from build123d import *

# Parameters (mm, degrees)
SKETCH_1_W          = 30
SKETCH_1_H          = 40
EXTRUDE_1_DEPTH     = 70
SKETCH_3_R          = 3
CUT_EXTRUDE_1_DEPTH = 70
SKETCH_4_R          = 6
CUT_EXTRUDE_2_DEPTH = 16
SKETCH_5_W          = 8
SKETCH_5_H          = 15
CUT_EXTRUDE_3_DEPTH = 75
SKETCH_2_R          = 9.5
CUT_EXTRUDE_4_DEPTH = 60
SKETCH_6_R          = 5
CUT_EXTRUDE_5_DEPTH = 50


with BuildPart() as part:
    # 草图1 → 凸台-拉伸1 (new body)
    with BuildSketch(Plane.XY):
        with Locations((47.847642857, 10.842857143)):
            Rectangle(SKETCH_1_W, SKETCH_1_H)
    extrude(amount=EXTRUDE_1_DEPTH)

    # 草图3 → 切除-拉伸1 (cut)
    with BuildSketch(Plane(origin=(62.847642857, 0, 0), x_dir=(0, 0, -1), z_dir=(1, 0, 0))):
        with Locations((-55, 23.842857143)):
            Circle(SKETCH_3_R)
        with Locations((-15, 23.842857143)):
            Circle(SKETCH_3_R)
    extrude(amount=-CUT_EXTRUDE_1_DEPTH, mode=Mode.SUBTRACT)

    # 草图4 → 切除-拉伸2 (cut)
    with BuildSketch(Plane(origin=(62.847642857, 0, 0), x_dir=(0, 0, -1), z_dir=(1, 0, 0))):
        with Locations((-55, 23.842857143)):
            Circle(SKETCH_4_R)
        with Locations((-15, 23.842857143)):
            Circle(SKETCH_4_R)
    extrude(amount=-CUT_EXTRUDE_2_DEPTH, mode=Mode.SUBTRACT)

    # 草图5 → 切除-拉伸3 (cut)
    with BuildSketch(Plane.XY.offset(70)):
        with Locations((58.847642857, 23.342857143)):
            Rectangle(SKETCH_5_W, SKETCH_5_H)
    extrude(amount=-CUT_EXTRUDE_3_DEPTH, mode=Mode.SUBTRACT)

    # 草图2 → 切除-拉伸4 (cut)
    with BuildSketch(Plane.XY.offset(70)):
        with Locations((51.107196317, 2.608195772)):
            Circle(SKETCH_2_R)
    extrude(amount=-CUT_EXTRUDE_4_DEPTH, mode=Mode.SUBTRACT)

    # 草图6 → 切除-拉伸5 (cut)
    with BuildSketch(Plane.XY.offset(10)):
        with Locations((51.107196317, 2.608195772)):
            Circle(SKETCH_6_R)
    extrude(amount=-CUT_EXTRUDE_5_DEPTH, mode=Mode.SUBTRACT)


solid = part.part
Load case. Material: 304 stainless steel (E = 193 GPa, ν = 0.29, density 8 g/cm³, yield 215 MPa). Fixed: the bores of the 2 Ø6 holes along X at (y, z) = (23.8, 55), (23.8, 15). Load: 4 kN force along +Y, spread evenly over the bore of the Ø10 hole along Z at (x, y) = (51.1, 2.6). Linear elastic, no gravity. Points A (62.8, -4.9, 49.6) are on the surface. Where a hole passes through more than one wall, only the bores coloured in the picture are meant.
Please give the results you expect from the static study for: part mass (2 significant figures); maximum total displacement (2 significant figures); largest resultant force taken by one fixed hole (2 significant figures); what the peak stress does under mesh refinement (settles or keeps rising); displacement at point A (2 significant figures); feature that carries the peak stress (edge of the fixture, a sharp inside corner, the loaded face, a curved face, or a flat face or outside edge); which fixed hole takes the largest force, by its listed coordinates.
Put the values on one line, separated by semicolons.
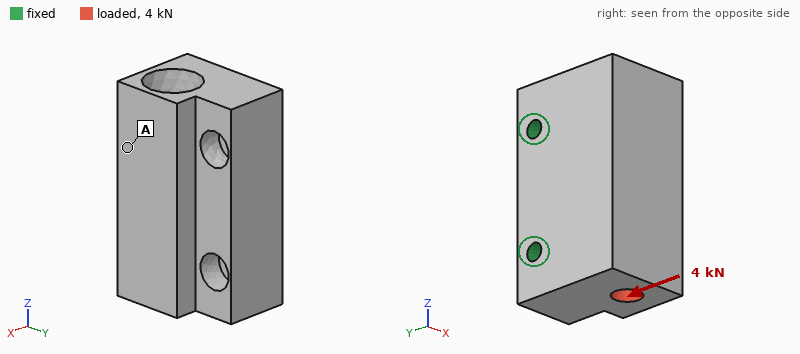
440 g; 12 µm; 4.7 kN; keeps rising; 6.0 µm; edge of the fixture; (23.8, 15)
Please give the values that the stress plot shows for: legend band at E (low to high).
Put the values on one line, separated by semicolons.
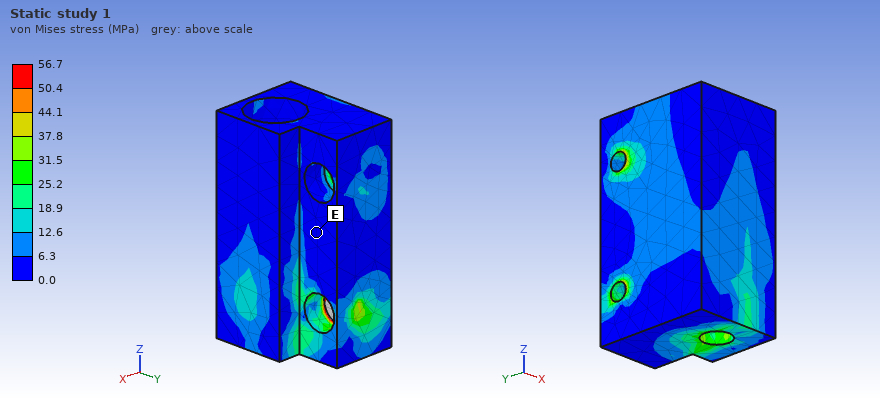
0.0 to 6.3 MPa
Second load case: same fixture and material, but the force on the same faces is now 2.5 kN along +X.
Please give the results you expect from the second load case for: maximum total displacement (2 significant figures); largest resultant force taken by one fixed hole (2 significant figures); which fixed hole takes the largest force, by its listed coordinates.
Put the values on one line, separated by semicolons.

13 µm; 2.8 kN; (23.8, 15)
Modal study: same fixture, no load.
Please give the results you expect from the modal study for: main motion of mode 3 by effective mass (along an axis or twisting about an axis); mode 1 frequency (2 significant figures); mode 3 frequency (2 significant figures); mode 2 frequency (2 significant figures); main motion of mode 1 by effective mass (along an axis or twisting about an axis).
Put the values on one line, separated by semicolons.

along Z; 5800 Hz; 12 kHz; 11 kHz; along X
